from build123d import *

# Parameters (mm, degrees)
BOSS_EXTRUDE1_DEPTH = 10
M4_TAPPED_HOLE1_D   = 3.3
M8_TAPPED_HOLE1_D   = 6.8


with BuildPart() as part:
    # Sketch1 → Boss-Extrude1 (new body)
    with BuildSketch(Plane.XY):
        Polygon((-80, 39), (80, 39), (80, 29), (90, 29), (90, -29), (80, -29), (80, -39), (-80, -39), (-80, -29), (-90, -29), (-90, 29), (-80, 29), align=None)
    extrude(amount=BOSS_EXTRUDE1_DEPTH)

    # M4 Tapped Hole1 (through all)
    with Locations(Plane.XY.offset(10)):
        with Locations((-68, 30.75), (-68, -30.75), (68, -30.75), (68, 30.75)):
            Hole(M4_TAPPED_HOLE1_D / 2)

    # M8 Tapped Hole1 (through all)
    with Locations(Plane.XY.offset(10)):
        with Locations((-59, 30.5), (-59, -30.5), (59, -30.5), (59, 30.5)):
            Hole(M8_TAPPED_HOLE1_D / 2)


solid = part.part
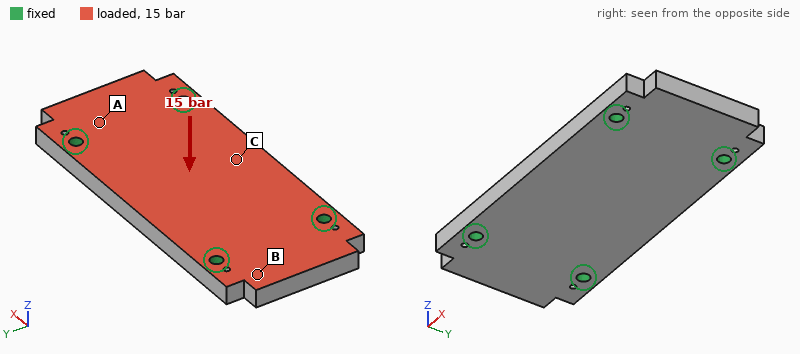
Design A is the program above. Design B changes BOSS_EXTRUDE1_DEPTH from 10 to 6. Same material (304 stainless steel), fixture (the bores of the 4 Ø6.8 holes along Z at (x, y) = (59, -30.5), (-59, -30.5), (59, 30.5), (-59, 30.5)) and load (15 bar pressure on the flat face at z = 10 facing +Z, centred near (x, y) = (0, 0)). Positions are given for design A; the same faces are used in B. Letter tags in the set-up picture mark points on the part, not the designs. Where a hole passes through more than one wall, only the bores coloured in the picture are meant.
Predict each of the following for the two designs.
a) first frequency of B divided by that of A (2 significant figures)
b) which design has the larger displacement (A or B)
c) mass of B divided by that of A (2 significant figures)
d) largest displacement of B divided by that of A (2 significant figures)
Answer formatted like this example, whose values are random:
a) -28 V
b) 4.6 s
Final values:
a) 0.64
b) B
c) 0.60
d) 4.2
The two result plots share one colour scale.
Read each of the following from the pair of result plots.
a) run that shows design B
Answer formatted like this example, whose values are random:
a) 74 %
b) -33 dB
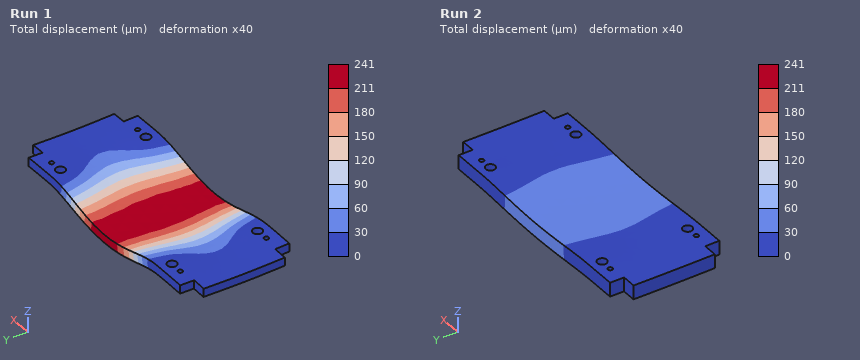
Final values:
a) Run 1
